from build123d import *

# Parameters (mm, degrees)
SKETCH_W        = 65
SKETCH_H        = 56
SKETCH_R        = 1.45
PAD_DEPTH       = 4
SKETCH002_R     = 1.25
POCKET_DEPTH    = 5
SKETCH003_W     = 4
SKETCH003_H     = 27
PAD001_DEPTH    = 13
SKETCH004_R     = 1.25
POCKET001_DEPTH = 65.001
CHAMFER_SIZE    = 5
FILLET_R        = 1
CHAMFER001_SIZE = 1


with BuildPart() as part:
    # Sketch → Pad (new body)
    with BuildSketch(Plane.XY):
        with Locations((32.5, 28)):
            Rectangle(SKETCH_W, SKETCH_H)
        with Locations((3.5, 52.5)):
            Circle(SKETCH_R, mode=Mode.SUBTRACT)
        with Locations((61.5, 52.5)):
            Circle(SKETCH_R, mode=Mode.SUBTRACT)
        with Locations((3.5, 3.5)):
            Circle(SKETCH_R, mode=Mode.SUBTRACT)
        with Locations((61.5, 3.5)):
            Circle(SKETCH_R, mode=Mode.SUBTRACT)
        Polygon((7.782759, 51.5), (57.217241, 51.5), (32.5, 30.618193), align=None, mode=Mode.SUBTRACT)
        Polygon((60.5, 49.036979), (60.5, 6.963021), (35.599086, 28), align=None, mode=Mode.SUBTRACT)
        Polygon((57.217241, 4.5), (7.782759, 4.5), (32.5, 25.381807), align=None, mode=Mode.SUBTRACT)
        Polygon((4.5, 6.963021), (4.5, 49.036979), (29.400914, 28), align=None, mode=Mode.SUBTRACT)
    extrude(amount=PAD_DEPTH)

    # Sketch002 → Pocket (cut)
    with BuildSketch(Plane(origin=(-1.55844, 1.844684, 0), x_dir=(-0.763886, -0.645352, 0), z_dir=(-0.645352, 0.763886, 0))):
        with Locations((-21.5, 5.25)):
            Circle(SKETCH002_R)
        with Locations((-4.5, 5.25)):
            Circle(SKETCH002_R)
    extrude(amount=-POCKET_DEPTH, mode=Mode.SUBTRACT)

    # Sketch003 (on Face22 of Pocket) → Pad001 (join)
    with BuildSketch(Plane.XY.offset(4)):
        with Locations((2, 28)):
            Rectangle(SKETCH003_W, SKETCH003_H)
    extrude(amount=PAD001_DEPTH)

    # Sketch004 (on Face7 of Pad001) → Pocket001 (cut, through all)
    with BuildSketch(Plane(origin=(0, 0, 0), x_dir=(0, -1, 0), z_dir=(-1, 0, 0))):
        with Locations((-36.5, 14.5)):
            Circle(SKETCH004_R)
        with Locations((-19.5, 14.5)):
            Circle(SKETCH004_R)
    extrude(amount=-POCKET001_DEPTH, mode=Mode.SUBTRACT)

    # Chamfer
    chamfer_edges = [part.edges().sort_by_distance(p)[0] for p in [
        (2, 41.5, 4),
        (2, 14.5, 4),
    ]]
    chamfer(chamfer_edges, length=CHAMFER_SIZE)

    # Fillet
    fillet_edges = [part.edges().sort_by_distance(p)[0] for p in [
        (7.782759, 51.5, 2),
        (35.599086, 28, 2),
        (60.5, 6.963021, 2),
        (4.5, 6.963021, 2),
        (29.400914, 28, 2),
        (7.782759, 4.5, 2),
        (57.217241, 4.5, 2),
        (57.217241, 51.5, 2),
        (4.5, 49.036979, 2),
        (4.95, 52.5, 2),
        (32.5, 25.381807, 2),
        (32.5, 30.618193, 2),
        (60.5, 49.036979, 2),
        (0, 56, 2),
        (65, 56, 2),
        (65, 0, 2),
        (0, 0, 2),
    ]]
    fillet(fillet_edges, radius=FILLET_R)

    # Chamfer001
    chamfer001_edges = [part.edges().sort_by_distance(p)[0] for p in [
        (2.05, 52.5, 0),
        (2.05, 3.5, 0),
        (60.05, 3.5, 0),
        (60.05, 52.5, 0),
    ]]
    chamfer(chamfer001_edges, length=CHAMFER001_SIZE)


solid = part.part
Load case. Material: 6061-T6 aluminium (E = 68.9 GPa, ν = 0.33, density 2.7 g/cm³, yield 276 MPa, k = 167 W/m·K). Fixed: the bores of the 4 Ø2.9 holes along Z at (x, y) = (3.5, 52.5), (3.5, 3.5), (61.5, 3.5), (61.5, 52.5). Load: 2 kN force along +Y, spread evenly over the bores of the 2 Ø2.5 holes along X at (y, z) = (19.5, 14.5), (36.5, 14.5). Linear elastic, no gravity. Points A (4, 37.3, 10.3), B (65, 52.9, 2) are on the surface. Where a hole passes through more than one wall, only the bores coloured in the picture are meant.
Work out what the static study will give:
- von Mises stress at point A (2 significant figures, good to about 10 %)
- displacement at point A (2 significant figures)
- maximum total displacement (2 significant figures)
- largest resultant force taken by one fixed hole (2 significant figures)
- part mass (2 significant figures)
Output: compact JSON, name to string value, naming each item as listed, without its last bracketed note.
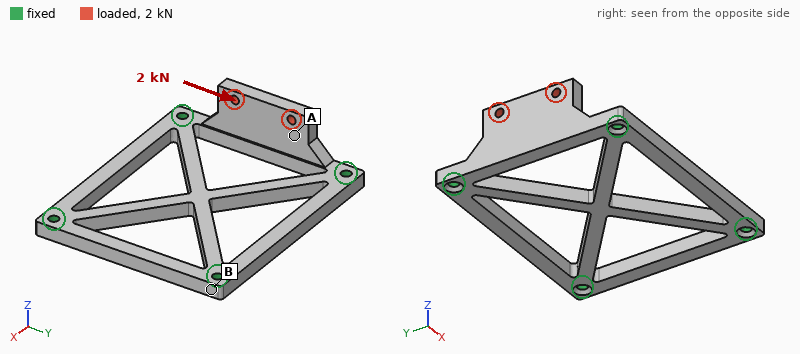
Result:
{"von Mises stress at point A": "50 MPa", "displacement at point A": "28 µm", "maximum total displacement": "48 µm", "largest resultant force taken by one fixed hole": "1.2 kN", "part mass": "21 g"}
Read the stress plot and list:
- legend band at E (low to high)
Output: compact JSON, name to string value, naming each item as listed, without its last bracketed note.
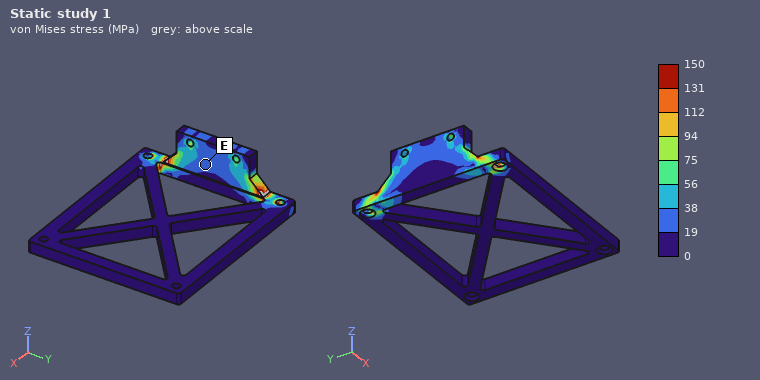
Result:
{"legend band at E": "19 to 38 MPa"}
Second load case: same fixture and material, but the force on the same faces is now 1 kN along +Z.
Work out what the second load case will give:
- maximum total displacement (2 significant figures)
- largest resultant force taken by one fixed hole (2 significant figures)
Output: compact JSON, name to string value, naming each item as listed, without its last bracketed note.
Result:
{"maximum total displacement": "49 µm", "largest resultant force taken by one fixed hole": "620 N"}
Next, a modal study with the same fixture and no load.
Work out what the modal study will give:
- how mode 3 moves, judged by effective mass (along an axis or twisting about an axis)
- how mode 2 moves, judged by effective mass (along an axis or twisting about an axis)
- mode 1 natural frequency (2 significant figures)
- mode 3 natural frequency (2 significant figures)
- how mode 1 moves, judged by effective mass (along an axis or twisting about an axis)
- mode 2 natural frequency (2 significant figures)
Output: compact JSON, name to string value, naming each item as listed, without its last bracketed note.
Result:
{"how mode 3 moves, judged by effective mass": "twisting about X", "how mode 2 moves, judged by effective mass": "along X", "mode 1 natural frequency": "4000 Hz", "mode 3 natural frequency": "6500 Hz", "how mode 1 moves, judged by effective mass": "along Z", "mode 2 natural frequency": "4500 Hz"}
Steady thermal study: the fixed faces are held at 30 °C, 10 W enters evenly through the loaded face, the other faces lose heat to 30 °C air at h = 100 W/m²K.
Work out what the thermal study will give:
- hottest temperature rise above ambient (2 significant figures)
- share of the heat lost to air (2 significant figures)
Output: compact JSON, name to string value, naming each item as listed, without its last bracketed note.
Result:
{"hottest temperature rise above ambient": "20 K", "share of the heat lost to air": "23 %"}
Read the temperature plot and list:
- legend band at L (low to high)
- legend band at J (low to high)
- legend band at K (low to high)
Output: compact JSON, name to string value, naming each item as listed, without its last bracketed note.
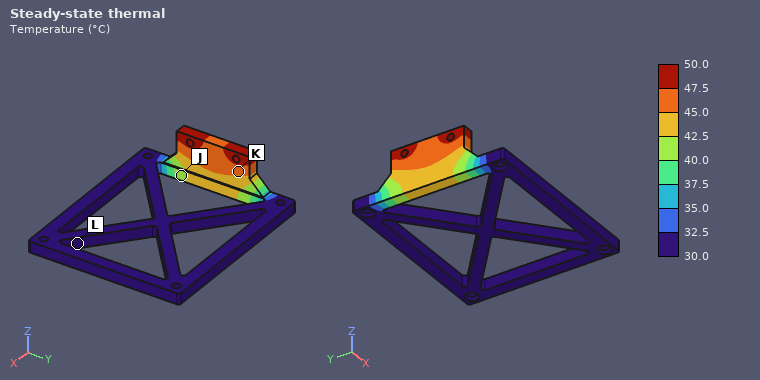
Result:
{"legend band at L": "30.0 to 32.5 °C", "legend band at J": "40.0 to 42.5 °C", "legend band at K": "45.0 to 47.5 °C"}
